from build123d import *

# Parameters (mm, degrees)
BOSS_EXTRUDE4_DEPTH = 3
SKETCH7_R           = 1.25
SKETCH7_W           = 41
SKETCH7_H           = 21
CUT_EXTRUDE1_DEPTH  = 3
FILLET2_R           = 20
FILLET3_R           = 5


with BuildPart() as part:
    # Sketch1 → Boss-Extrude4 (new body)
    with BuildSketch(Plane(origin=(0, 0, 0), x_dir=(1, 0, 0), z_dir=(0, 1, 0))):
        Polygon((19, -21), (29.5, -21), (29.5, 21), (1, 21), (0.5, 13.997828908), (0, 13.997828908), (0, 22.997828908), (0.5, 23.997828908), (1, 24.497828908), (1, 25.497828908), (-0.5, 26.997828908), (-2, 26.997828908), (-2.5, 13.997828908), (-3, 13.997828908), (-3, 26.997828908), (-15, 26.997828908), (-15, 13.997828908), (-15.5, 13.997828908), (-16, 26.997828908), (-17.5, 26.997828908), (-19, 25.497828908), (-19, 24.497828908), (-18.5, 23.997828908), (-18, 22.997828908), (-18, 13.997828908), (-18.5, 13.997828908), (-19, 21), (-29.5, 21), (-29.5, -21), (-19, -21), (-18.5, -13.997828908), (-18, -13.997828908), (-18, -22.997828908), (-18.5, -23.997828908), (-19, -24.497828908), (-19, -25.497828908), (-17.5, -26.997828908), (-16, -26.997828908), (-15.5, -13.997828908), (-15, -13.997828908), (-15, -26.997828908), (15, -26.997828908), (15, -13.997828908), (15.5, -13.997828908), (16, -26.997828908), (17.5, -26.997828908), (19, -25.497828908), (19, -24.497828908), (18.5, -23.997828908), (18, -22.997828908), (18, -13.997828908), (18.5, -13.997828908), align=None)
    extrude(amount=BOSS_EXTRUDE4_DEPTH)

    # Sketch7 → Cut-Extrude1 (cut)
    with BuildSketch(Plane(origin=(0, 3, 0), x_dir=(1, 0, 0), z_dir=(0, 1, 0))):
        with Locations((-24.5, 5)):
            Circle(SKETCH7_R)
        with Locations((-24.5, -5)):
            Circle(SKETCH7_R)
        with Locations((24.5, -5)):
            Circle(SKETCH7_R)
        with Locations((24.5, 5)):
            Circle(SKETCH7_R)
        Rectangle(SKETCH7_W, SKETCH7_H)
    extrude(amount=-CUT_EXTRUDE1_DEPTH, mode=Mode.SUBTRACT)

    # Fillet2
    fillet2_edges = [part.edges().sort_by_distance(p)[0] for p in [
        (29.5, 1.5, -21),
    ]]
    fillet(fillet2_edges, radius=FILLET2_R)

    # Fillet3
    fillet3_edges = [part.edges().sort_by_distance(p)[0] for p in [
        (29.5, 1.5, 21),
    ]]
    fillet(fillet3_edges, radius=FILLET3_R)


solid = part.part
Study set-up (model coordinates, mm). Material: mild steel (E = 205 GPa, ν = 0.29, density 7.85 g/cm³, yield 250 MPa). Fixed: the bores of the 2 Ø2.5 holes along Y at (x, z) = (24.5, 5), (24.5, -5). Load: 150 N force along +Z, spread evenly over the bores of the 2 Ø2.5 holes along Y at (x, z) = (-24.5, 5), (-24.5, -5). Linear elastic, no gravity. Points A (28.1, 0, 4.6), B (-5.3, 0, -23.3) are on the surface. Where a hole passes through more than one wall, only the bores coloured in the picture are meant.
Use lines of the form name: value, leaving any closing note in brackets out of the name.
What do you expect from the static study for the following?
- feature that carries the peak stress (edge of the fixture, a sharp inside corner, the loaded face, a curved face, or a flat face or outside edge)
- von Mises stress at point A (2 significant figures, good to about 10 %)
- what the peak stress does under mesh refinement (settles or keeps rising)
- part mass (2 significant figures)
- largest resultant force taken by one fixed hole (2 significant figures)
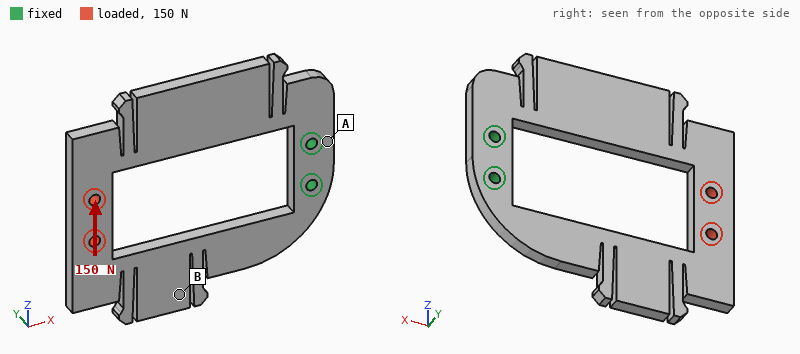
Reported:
feature that carries the peak stress: a sharp inside corner
von Mises stress at point A: 32 MPa
what the peak stress does under mesh refinement: keeps rising
part mass: 42 g
largest resultant force taken by one fixed hole: 460 N
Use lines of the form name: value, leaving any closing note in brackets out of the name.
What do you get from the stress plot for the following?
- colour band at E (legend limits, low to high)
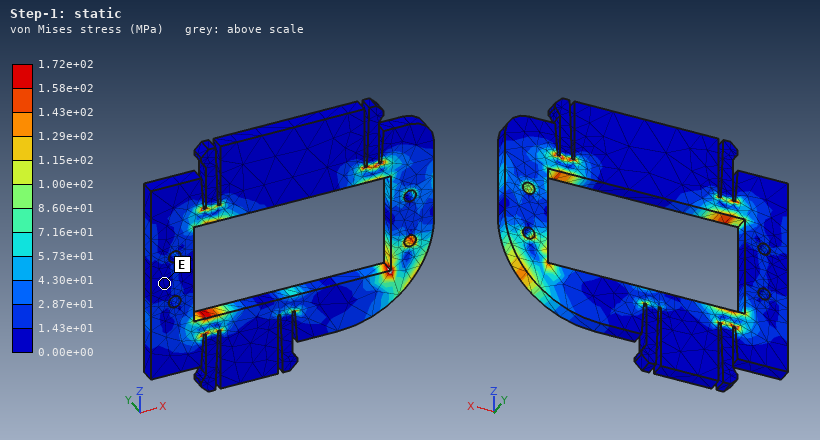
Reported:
colour band at E: 0.00e+00 to 1.43e+01 MPa
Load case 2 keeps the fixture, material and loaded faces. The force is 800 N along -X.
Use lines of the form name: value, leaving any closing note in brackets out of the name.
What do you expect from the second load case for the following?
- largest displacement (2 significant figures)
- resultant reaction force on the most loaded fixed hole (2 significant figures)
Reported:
largest displacement: 19 µm
resultant reaction force on the most loaded fixed hole: 410 N
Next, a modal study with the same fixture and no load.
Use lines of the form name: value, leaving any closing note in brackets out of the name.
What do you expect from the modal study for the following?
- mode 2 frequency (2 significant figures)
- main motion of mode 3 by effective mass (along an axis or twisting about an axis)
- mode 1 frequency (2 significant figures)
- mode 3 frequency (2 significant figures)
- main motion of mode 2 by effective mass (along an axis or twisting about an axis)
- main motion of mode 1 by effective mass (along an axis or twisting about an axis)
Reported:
mode 2 frequency: 940 Hz
main motion of mode 3 by effective mass: along Z
mode 1 frequency: 470 Hz
mode 3 frequency: 1200 Hz
main motion of mode 2 by effective mass: twisting about X
main motion of mode 1 by effective mass: along Y
